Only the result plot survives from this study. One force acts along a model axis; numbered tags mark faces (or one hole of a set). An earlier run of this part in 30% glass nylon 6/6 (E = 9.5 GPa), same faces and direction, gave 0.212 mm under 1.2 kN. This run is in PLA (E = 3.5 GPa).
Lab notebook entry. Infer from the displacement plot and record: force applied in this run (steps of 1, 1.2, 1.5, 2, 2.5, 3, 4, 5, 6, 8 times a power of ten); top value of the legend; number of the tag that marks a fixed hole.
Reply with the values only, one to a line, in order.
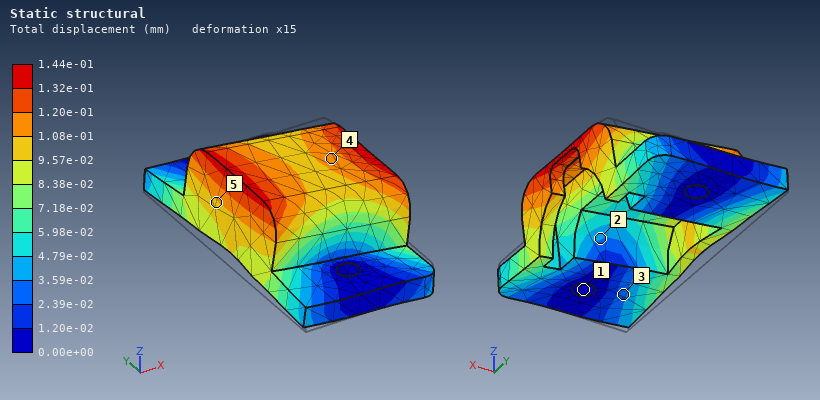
300 N
1.44e-01 mm
1
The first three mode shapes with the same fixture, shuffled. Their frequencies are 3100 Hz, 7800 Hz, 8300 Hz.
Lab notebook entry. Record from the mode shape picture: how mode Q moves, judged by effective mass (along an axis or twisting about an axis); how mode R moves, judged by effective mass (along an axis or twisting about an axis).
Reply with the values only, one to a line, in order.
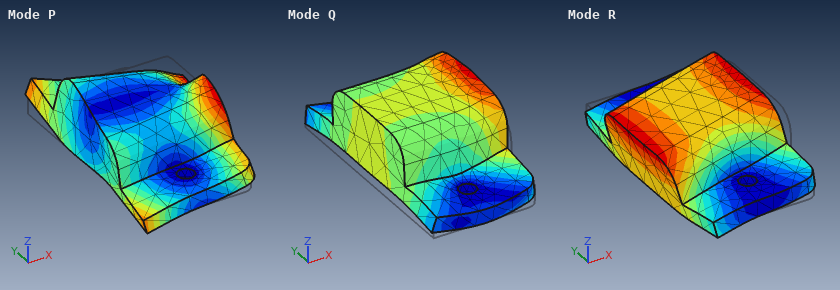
along Z
along X
